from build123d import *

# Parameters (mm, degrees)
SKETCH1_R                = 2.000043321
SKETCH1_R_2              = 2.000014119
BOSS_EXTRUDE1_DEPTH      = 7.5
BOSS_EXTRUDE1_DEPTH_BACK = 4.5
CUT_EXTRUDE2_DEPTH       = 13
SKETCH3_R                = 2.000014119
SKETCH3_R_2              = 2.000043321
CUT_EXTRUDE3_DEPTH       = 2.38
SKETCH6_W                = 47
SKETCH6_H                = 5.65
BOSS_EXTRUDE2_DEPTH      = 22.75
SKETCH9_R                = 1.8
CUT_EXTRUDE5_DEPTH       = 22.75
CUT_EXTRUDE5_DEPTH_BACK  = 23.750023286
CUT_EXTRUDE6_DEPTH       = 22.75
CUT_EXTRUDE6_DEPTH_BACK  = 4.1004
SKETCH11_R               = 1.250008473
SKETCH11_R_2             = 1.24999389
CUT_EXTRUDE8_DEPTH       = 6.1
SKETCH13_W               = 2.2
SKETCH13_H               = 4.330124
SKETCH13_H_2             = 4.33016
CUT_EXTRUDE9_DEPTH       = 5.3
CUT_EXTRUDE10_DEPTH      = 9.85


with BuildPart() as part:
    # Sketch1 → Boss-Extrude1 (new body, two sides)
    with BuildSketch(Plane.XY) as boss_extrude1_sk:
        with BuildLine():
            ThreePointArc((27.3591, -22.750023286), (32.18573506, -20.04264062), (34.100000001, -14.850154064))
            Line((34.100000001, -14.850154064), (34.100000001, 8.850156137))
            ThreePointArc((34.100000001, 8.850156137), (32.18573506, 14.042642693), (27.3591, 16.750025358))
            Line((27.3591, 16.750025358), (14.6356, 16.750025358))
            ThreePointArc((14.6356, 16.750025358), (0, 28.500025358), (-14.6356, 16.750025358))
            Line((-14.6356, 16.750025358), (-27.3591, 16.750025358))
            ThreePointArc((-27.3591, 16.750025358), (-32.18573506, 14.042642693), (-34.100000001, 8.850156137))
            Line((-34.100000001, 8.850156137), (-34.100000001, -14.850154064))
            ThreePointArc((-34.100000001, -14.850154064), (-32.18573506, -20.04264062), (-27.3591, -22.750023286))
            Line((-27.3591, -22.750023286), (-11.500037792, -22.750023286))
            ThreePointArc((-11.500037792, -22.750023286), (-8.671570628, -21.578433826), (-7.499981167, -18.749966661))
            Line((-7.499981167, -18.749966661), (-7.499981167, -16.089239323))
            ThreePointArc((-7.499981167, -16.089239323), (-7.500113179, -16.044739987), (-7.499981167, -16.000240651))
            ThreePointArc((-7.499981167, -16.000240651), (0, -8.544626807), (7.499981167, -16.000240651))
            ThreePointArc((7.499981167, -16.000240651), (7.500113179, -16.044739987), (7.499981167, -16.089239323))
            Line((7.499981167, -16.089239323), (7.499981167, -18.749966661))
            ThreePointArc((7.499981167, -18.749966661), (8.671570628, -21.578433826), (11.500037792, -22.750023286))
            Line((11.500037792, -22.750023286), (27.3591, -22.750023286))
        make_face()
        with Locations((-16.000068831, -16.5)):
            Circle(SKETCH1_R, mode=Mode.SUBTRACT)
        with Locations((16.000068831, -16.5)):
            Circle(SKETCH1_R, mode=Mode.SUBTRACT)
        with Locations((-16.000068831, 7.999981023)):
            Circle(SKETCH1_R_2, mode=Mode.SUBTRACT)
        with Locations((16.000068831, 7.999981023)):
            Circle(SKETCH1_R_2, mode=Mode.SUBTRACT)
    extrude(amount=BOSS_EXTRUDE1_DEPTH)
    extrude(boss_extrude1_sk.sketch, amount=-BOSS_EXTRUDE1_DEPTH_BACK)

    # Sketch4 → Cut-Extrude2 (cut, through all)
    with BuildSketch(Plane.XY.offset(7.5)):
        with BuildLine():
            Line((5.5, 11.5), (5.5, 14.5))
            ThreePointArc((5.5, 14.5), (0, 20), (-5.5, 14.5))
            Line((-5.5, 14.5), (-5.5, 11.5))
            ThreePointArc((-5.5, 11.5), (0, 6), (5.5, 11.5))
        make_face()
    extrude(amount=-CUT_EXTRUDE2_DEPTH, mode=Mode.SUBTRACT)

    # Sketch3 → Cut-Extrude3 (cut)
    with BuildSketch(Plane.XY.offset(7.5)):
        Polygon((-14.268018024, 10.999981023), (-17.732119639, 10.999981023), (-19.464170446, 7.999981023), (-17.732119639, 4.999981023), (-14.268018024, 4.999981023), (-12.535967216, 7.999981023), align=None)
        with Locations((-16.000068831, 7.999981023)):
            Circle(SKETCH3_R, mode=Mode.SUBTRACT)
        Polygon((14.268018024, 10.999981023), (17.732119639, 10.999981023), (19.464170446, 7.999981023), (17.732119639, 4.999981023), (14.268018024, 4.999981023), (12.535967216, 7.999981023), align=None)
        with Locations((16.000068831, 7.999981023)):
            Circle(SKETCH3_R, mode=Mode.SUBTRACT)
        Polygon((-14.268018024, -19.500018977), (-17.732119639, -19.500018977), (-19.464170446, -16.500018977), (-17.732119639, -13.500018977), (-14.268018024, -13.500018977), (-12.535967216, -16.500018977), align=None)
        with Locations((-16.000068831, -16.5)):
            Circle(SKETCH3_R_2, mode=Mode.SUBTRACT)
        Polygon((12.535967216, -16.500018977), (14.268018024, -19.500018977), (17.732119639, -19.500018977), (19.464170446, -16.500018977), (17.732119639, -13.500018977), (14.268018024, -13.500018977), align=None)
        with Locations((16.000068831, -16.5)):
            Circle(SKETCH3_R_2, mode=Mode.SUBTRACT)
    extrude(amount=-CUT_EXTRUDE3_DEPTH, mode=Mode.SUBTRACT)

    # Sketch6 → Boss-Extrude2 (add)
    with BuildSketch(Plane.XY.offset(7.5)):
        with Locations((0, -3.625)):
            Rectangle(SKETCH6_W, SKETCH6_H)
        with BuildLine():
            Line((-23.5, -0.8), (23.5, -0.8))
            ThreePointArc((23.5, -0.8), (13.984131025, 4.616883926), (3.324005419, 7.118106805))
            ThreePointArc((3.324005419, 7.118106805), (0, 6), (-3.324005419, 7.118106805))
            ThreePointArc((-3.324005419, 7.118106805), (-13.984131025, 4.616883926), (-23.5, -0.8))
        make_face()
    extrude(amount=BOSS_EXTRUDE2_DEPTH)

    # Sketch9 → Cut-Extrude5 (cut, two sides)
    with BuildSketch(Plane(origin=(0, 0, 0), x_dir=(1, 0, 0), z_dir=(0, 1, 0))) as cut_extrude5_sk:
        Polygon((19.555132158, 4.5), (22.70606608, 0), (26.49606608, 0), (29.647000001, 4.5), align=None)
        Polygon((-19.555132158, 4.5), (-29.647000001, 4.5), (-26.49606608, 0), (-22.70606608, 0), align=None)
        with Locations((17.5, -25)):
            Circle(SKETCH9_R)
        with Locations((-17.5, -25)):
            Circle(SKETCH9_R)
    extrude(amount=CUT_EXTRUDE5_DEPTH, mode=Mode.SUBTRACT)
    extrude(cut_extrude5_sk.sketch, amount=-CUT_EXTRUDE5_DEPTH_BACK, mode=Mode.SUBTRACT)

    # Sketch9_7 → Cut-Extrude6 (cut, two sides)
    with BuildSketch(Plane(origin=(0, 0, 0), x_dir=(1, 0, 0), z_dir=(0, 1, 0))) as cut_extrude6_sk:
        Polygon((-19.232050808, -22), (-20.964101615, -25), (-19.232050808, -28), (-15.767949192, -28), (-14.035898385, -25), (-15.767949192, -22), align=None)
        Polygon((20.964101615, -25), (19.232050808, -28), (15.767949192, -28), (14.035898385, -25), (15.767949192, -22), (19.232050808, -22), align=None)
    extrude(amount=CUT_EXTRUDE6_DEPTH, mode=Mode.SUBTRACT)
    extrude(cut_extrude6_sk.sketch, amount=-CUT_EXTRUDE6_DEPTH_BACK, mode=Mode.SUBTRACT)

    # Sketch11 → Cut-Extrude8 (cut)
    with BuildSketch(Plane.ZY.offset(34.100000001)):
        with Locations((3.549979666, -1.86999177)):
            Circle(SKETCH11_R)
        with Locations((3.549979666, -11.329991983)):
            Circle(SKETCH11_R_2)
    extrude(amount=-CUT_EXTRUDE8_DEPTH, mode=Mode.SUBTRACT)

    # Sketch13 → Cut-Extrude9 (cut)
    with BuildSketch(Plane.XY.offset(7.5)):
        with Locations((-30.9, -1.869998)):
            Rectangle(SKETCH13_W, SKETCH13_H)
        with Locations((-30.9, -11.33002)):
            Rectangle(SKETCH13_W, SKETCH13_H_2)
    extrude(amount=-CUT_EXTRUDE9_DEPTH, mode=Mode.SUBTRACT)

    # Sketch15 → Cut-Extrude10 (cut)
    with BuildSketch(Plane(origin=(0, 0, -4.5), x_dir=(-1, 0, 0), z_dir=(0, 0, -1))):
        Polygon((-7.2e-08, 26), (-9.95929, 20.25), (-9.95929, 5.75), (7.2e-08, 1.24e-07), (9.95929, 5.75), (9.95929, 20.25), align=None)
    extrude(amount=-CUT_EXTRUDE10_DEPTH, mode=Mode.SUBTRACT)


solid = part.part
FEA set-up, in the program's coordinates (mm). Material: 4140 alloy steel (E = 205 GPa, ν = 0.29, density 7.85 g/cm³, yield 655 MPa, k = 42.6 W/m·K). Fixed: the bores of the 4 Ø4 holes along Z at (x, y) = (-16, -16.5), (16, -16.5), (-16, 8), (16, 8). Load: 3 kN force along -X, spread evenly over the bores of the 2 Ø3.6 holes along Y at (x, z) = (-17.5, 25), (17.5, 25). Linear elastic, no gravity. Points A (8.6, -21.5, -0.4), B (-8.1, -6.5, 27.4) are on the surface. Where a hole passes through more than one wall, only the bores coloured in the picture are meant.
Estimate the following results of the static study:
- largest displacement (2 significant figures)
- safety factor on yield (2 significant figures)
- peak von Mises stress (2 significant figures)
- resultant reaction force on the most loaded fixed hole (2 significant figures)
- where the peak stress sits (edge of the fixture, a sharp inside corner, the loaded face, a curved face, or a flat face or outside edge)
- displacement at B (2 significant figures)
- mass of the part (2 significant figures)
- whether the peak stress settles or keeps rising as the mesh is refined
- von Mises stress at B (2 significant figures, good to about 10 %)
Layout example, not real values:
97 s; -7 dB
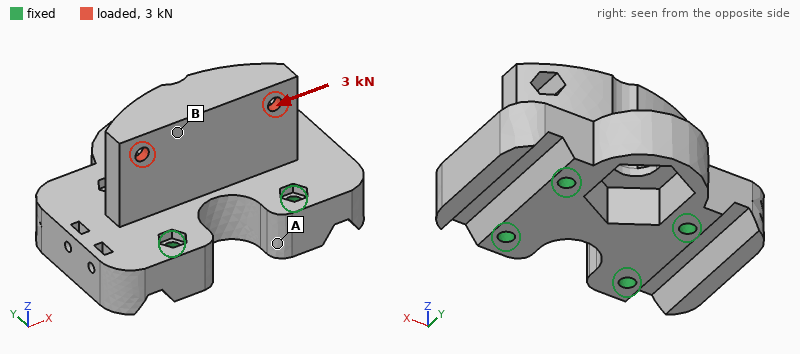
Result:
8.2 µm; 5.5; 120 MPa; 1.7 kN; the loaded face; 4.7 µm; 280 g; settles; 21 MPa
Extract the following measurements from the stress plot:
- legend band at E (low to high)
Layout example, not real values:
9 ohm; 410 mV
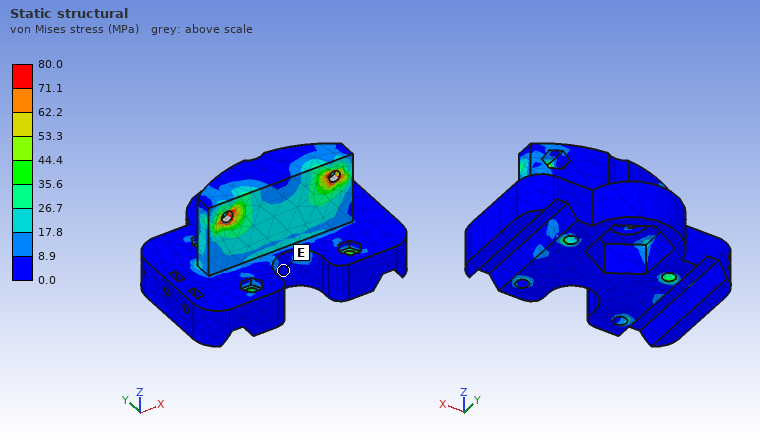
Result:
0.0 to 8.9 MPa
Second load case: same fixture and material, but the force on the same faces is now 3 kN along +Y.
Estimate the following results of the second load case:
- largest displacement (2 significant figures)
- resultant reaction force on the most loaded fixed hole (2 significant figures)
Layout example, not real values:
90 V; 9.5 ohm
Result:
20 µm; 1.7 kN
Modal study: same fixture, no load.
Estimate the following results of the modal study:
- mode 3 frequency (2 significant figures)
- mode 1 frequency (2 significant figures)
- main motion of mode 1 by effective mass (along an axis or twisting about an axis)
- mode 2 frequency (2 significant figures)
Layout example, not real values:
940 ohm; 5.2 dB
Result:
17 kHz; 11 kHz; along Y; 15 kHz
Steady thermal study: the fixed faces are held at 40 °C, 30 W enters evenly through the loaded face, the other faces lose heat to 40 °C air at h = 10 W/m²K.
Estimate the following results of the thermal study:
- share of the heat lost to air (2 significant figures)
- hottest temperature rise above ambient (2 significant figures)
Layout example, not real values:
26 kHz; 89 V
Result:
4.6 %; 74 K
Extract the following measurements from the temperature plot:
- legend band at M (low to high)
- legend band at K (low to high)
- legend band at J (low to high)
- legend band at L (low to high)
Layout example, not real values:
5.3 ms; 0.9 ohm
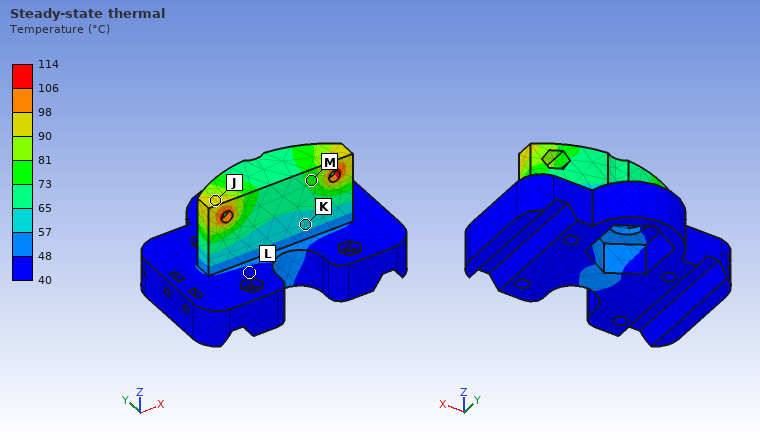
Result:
73 to 81 °C; 57 to 65 °C; 90 to 98 °C; 40 to 48 °C
